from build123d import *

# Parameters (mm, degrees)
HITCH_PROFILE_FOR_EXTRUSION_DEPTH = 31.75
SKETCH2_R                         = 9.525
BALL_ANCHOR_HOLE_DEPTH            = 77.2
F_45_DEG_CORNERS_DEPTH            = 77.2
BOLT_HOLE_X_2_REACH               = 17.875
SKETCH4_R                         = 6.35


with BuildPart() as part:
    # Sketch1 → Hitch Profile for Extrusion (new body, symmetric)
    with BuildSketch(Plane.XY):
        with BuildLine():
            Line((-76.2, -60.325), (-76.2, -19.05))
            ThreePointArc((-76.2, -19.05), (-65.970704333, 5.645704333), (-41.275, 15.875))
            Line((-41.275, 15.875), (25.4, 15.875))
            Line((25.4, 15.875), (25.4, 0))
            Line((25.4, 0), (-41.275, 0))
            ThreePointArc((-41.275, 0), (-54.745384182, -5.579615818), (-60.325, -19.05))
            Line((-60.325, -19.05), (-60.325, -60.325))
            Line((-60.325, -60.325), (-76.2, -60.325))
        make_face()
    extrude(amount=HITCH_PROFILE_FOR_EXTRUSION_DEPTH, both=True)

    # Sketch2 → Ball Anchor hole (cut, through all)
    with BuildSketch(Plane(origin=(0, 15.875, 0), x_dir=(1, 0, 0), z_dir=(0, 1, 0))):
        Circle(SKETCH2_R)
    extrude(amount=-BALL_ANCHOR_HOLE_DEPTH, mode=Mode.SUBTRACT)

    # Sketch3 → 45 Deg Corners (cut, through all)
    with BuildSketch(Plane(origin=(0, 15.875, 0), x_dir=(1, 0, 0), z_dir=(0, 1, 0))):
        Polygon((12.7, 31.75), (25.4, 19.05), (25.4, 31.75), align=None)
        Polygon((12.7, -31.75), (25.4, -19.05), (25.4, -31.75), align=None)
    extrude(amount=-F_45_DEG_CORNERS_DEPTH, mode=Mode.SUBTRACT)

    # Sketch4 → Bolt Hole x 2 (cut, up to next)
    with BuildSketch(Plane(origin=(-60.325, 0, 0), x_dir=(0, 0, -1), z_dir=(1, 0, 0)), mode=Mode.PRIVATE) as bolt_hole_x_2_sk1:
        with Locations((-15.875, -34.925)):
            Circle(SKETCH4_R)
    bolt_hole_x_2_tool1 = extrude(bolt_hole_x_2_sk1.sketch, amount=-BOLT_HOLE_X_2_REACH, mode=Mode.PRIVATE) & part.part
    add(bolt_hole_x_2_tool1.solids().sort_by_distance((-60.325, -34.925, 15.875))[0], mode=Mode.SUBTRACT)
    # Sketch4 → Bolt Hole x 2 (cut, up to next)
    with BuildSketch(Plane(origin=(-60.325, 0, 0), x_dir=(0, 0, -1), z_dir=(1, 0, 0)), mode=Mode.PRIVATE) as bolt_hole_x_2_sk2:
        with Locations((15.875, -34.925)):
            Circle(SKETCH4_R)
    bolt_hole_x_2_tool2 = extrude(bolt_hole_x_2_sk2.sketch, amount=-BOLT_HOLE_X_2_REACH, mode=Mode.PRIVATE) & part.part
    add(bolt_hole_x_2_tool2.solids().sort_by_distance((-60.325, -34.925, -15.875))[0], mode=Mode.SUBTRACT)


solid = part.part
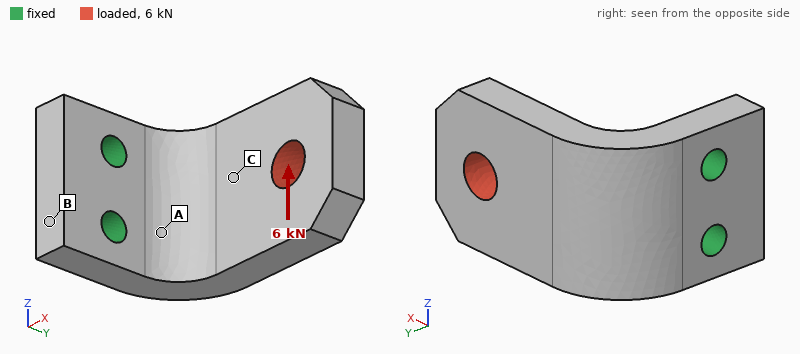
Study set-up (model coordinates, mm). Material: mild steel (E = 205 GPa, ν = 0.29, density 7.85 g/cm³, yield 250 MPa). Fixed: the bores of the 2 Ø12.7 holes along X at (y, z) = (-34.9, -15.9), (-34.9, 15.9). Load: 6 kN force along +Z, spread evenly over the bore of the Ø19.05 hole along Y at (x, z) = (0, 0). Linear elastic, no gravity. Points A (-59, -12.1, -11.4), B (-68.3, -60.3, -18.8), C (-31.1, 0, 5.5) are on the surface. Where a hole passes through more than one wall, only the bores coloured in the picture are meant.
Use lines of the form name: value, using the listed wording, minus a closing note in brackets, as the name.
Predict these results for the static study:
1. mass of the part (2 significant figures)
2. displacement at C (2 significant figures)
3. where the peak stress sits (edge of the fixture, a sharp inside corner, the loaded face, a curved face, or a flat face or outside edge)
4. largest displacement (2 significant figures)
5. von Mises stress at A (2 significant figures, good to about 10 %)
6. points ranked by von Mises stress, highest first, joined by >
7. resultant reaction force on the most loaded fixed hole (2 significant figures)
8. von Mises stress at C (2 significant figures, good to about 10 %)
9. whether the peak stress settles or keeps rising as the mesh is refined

mass of the part: 1.1 kg
displacement at C: 0.055 mm
where the peak stress sits: edge of the fixture
largest displacement: 0.15 mm
von Mises stress at A: 100 MPa
points ranked by von Mises stress, highest first, joined by >: A > C > B
resultant reaction force on the most loaded fixed hole: 11 kN
von Mises stress at C: 30 MPa
whether the peak stress settles or keeps rising as the mesh is refined: keeps rising
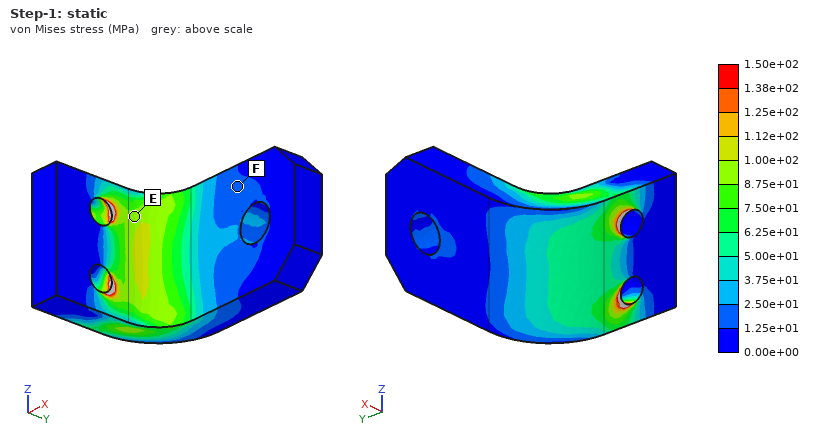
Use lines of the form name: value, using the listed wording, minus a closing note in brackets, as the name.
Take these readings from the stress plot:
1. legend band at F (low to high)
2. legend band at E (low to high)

legend band at F: 1.25e+01 to 2.50e+01 MPa
legend band at E: 8.75e+01 to 1.00e+02 MPa
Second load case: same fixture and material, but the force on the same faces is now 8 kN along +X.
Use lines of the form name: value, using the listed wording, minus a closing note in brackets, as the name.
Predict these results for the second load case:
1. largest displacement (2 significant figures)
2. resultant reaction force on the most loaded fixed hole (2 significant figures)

largest displacement: 0.16 mm
resultant reaction force on the most loaded fixed hole: 4.0 kN
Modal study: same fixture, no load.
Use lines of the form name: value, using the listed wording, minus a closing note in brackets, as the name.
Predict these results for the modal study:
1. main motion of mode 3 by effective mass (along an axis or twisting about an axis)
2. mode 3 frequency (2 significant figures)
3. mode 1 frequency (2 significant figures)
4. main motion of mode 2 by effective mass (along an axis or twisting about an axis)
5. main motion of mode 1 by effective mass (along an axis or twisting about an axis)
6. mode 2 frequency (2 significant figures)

main motion of mode 3 by effective mass: along X
mode 3 frequency: 3900 Hz
mode 1 frequency: 1100 Hz
main motion of mode 2 by effective mass: along Z
main motion of mode 1 by effective mass: along Y
mode 2 frequency: 1900 Hz
